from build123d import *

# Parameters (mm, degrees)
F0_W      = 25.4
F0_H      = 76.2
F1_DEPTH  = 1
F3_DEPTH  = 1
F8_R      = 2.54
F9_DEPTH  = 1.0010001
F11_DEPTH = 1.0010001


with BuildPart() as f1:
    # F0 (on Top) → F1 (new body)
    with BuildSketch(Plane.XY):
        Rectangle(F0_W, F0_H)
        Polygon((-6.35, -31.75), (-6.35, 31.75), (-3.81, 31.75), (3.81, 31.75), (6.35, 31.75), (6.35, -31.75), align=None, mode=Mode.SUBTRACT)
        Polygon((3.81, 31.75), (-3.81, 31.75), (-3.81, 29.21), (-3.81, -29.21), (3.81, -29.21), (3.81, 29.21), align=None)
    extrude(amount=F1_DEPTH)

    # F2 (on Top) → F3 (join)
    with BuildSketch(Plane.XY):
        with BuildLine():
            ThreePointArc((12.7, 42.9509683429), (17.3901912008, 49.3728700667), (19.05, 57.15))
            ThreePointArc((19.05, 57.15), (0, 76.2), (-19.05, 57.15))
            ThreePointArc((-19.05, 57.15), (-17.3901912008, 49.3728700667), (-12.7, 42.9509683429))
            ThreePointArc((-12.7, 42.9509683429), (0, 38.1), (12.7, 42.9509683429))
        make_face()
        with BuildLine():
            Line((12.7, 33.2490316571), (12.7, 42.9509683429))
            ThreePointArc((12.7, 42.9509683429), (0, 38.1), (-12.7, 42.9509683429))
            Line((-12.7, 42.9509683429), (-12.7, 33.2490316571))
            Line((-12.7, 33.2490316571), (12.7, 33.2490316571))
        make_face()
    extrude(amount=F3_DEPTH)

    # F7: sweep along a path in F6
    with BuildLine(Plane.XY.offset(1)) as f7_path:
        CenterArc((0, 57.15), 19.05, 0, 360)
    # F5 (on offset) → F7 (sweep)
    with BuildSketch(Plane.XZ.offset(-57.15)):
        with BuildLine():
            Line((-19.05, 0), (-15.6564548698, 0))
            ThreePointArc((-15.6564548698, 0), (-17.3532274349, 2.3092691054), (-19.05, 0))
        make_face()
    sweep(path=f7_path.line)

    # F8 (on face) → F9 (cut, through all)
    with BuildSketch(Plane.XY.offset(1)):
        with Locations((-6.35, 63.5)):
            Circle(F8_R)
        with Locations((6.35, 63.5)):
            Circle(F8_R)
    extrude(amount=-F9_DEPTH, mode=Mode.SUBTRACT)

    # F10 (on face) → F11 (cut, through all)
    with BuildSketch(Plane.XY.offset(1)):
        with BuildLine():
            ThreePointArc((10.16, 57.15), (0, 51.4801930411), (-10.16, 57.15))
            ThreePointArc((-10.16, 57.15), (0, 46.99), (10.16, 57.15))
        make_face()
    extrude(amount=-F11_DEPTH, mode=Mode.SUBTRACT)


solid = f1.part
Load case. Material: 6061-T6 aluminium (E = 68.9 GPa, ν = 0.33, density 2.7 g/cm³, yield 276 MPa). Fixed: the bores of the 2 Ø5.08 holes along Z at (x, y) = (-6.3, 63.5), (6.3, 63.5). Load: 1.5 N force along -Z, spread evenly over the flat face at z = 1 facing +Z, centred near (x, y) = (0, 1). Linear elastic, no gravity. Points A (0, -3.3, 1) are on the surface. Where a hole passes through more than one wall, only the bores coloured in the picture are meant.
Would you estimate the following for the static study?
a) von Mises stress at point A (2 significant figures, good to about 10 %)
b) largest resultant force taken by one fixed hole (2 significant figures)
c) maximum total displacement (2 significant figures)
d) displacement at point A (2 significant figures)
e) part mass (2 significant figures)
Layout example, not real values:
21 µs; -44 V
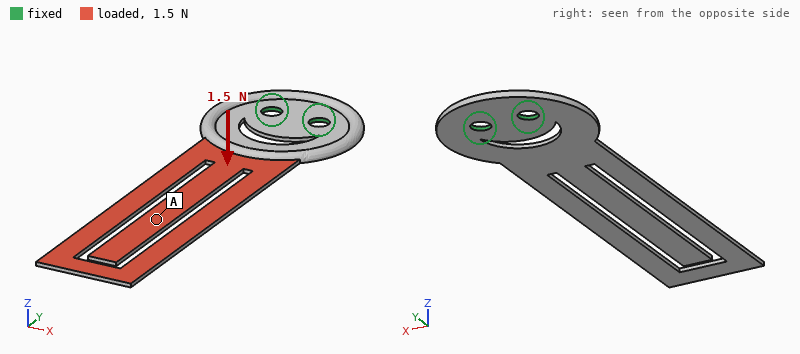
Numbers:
1.9 MPa; 4.4 N; 1.2 mm; 0.48 mm; 8.1 g
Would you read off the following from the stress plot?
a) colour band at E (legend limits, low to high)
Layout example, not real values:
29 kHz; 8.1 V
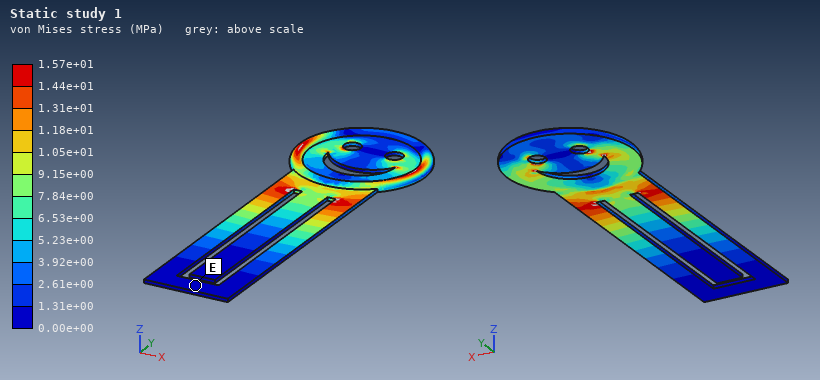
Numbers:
0.00e+00 to 1.31e+00 MPa
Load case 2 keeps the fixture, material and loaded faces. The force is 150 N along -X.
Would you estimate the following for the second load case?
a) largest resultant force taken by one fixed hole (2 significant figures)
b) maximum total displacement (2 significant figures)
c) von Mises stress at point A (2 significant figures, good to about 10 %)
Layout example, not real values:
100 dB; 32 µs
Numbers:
510 N; 0.81 mm; 12 MPa
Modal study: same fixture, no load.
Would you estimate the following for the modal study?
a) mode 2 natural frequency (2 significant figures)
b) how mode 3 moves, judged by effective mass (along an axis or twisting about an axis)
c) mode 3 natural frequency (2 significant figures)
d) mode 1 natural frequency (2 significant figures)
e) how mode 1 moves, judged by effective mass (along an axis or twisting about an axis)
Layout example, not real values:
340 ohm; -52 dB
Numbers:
180 Hz; twisting about Y; 540 Hz; 100 Hz; along Z
